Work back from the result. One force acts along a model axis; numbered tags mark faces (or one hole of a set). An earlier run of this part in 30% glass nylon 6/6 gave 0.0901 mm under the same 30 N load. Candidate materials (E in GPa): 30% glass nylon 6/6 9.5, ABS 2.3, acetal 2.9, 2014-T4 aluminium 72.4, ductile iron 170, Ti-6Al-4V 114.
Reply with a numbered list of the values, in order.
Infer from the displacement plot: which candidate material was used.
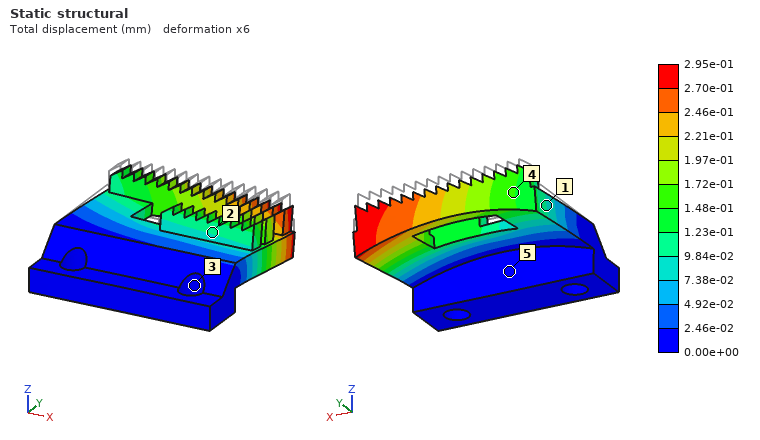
1. acetal
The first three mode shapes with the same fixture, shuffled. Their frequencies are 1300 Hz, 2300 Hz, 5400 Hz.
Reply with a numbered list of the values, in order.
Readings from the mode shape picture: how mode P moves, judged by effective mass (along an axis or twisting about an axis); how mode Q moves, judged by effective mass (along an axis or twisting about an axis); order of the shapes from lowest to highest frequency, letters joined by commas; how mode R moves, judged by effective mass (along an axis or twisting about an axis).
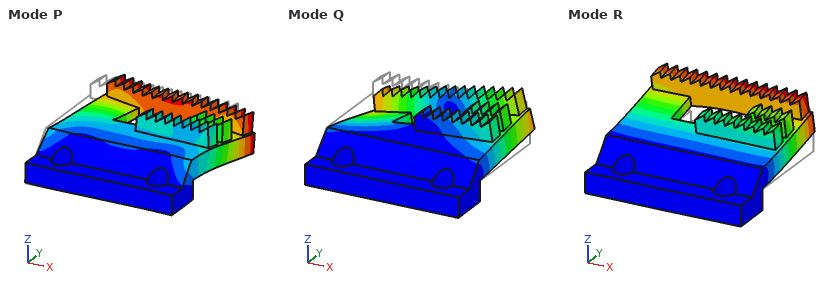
1. along X
2. twisting about Y
3. R, Q, P
4. along Z
